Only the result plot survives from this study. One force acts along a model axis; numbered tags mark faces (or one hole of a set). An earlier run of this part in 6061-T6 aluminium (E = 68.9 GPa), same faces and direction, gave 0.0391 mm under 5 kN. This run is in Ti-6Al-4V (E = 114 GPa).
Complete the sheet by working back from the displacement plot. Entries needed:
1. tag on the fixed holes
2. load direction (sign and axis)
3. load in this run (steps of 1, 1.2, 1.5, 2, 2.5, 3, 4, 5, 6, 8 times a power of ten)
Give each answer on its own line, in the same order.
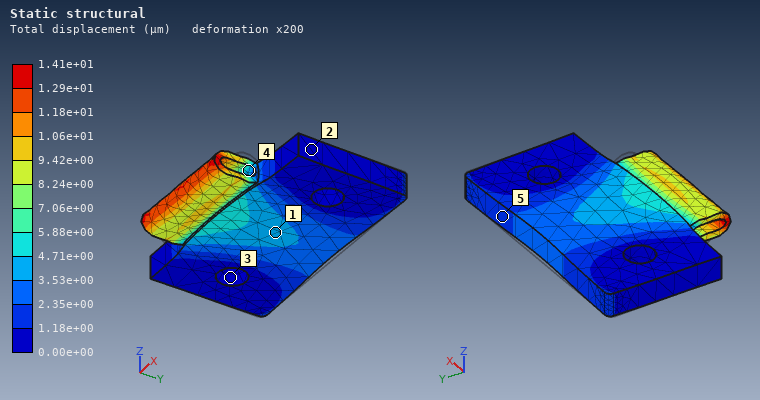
3
-Y
3 kN
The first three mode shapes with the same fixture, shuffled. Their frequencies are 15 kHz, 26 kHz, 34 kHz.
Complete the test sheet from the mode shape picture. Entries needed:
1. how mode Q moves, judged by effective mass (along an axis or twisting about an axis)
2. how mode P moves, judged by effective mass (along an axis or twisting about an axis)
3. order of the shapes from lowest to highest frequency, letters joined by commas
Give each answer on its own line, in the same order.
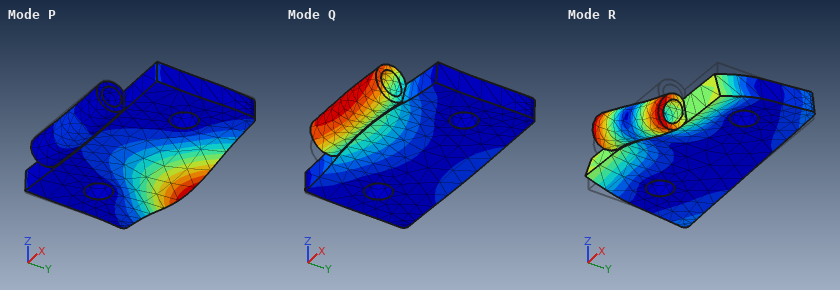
along Z
along Z
Q, P, R
